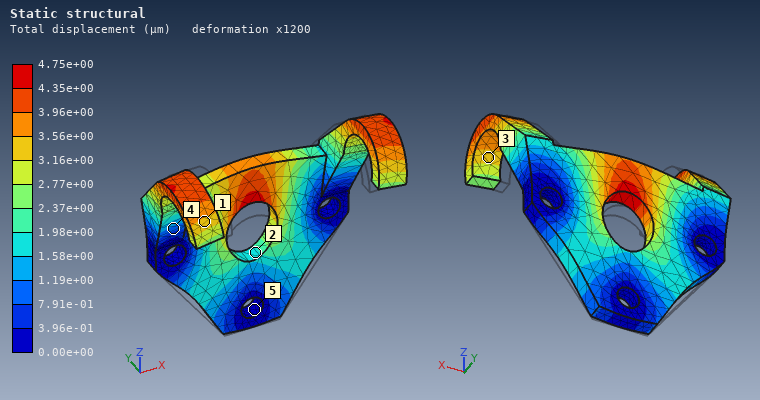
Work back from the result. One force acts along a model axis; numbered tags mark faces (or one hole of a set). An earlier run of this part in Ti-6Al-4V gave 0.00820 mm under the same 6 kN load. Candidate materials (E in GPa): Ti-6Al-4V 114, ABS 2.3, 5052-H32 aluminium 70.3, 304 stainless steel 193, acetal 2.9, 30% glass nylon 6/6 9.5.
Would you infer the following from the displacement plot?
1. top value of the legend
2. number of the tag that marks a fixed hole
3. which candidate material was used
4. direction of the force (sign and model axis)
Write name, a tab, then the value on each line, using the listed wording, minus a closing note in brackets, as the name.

top value of the legend	4.75e+00 µm
number of the tag that marks a fixed hole	5
which candidate material was used	304 stainless steel
direction of the force	+Z
